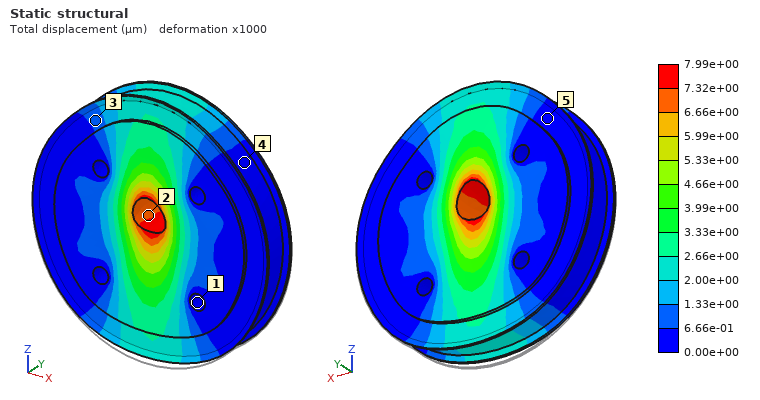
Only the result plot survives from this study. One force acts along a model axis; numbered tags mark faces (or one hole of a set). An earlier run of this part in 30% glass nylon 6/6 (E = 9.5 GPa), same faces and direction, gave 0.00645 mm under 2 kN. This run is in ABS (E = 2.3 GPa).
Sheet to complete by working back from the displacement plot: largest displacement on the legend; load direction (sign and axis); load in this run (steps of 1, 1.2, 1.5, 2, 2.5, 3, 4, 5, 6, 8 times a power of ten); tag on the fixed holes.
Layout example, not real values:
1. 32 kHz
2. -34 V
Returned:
1. 7.99e+00 µm
2. +Z
3. 600 N
4. 1
